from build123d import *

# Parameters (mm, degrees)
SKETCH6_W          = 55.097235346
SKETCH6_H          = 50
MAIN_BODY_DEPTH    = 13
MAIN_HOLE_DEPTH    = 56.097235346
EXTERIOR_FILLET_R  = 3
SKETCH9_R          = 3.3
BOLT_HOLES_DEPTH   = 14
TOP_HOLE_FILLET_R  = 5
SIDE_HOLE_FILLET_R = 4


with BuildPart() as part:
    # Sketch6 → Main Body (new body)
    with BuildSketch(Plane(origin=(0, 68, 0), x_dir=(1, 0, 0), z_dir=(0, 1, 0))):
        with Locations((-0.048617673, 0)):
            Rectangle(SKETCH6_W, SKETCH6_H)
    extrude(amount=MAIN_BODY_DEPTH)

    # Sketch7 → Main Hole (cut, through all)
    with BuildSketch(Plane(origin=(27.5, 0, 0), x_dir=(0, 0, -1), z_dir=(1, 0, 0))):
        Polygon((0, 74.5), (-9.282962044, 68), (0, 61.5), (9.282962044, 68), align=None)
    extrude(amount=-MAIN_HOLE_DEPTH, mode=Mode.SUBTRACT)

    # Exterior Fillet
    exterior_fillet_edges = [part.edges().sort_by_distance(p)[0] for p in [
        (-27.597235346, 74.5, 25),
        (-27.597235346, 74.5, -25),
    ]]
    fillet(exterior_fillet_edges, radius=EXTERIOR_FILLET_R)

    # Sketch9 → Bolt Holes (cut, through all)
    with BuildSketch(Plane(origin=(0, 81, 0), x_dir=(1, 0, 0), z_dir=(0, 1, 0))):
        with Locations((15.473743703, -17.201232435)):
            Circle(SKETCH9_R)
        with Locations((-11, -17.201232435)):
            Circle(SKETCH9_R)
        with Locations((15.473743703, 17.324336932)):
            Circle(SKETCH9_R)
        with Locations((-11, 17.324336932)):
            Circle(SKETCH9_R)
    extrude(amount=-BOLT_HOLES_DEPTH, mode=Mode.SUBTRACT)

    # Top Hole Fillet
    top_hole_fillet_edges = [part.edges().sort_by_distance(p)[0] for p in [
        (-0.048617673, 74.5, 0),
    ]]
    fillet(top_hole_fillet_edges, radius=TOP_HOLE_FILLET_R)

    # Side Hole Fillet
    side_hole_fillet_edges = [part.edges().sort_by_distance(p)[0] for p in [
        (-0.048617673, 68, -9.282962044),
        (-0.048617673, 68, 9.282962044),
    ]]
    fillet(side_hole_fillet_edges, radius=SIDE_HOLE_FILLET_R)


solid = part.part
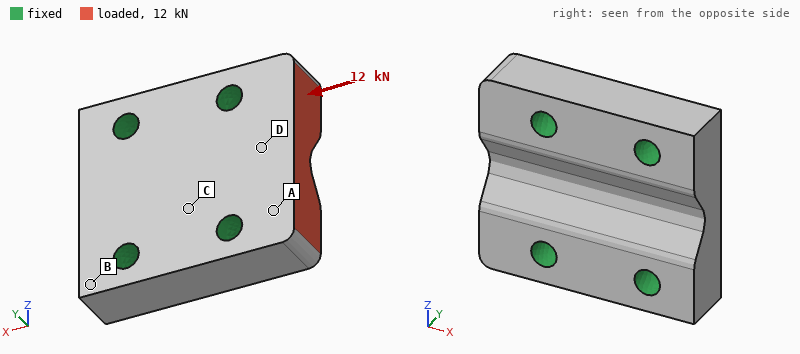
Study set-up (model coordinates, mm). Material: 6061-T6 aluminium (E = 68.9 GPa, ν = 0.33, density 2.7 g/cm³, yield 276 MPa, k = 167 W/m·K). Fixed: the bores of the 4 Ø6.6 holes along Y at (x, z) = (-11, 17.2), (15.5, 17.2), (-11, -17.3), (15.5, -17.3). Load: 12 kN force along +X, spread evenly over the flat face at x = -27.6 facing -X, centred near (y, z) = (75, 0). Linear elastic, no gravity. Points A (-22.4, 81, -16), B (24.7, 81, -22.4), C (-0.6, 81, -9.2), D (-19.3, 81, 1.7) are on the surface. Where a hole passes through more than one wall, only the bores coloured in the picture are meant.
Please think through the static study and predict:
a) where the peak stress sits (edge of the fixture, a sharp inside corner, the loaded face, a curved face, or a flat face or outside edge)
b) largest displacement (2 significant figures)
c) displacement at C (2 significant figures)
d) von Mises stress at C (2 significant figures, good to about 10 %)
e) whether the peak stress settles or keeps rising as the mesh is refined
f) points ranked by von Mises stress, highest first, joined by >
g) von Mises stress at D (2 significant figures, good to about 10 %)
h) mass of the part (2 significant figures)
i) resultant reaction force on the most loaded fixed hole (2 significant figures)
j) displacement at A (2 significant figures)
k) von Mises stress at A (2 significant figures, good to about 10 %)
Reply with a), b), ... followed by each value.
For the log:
a) edge of the fixture
b) 9.1 µm
c) 1.6 µm
d) 10 MPa
e) keeps rising
f) A > D > C > B
g) 17 MPa
h) 83 g
i) 5.3 kN
j) 3.9 µm
k) 26 MPa
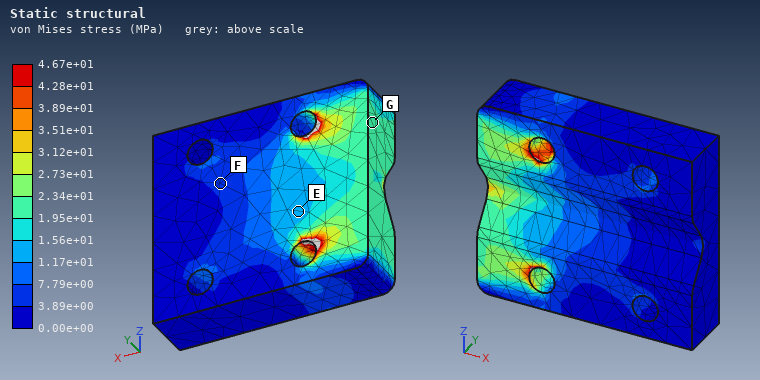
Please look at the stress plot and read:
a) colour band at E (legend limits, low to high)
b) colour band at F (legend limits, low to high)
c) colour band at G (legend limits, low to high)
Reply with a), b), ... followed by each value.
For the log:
a) 1.17e+01 to 1.56e+01 MPa
b) 3.89e+00 to 7.79e+00 MPa
c) 1.95e+01 to 2.34e+01 MPa
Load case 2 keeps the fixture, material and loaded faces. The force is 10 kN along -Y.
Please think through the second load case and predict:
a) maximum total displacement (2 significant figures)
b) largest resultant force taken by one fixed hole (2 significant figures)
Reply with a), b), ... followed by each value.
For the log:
a) 58 µm
b) 5.6 kN
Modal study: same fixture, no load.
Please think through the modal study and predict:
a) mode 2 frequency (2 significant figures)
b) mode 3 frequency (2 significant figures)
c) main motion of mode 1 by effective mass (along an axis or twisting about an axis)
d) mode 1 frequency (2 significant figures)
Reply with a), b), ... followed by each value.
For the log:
a) 34 kHz
b) 34 kHz
c) along Y
d) 26 kHz
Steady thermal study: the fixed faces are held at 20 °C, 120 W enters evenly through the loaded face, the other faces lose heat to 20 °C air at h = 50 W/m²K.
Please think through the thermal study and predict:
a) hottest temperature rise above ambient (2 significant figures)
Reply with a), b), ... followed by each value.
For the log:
a) 24 K
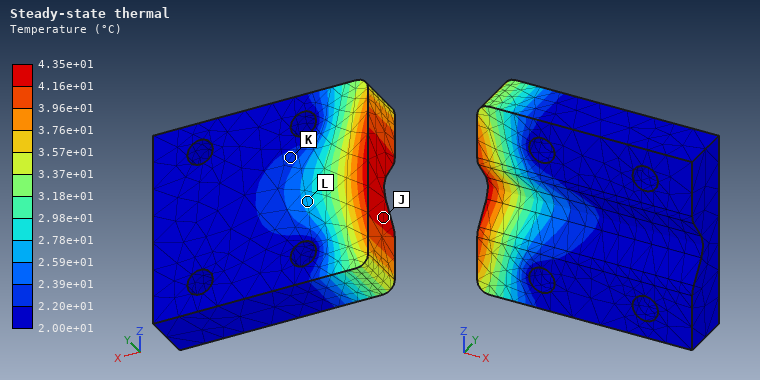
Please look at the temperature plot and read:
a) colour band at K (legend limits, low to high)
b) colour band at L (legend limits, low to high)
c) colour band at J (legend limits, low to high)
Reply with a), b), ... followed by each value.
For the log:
a) 2.20e+01 to 2.39e+01 °C
b) 2.59e+01 to 2.78e+01 °C
c) 4.16e+01 to 4.35e+01 °C
